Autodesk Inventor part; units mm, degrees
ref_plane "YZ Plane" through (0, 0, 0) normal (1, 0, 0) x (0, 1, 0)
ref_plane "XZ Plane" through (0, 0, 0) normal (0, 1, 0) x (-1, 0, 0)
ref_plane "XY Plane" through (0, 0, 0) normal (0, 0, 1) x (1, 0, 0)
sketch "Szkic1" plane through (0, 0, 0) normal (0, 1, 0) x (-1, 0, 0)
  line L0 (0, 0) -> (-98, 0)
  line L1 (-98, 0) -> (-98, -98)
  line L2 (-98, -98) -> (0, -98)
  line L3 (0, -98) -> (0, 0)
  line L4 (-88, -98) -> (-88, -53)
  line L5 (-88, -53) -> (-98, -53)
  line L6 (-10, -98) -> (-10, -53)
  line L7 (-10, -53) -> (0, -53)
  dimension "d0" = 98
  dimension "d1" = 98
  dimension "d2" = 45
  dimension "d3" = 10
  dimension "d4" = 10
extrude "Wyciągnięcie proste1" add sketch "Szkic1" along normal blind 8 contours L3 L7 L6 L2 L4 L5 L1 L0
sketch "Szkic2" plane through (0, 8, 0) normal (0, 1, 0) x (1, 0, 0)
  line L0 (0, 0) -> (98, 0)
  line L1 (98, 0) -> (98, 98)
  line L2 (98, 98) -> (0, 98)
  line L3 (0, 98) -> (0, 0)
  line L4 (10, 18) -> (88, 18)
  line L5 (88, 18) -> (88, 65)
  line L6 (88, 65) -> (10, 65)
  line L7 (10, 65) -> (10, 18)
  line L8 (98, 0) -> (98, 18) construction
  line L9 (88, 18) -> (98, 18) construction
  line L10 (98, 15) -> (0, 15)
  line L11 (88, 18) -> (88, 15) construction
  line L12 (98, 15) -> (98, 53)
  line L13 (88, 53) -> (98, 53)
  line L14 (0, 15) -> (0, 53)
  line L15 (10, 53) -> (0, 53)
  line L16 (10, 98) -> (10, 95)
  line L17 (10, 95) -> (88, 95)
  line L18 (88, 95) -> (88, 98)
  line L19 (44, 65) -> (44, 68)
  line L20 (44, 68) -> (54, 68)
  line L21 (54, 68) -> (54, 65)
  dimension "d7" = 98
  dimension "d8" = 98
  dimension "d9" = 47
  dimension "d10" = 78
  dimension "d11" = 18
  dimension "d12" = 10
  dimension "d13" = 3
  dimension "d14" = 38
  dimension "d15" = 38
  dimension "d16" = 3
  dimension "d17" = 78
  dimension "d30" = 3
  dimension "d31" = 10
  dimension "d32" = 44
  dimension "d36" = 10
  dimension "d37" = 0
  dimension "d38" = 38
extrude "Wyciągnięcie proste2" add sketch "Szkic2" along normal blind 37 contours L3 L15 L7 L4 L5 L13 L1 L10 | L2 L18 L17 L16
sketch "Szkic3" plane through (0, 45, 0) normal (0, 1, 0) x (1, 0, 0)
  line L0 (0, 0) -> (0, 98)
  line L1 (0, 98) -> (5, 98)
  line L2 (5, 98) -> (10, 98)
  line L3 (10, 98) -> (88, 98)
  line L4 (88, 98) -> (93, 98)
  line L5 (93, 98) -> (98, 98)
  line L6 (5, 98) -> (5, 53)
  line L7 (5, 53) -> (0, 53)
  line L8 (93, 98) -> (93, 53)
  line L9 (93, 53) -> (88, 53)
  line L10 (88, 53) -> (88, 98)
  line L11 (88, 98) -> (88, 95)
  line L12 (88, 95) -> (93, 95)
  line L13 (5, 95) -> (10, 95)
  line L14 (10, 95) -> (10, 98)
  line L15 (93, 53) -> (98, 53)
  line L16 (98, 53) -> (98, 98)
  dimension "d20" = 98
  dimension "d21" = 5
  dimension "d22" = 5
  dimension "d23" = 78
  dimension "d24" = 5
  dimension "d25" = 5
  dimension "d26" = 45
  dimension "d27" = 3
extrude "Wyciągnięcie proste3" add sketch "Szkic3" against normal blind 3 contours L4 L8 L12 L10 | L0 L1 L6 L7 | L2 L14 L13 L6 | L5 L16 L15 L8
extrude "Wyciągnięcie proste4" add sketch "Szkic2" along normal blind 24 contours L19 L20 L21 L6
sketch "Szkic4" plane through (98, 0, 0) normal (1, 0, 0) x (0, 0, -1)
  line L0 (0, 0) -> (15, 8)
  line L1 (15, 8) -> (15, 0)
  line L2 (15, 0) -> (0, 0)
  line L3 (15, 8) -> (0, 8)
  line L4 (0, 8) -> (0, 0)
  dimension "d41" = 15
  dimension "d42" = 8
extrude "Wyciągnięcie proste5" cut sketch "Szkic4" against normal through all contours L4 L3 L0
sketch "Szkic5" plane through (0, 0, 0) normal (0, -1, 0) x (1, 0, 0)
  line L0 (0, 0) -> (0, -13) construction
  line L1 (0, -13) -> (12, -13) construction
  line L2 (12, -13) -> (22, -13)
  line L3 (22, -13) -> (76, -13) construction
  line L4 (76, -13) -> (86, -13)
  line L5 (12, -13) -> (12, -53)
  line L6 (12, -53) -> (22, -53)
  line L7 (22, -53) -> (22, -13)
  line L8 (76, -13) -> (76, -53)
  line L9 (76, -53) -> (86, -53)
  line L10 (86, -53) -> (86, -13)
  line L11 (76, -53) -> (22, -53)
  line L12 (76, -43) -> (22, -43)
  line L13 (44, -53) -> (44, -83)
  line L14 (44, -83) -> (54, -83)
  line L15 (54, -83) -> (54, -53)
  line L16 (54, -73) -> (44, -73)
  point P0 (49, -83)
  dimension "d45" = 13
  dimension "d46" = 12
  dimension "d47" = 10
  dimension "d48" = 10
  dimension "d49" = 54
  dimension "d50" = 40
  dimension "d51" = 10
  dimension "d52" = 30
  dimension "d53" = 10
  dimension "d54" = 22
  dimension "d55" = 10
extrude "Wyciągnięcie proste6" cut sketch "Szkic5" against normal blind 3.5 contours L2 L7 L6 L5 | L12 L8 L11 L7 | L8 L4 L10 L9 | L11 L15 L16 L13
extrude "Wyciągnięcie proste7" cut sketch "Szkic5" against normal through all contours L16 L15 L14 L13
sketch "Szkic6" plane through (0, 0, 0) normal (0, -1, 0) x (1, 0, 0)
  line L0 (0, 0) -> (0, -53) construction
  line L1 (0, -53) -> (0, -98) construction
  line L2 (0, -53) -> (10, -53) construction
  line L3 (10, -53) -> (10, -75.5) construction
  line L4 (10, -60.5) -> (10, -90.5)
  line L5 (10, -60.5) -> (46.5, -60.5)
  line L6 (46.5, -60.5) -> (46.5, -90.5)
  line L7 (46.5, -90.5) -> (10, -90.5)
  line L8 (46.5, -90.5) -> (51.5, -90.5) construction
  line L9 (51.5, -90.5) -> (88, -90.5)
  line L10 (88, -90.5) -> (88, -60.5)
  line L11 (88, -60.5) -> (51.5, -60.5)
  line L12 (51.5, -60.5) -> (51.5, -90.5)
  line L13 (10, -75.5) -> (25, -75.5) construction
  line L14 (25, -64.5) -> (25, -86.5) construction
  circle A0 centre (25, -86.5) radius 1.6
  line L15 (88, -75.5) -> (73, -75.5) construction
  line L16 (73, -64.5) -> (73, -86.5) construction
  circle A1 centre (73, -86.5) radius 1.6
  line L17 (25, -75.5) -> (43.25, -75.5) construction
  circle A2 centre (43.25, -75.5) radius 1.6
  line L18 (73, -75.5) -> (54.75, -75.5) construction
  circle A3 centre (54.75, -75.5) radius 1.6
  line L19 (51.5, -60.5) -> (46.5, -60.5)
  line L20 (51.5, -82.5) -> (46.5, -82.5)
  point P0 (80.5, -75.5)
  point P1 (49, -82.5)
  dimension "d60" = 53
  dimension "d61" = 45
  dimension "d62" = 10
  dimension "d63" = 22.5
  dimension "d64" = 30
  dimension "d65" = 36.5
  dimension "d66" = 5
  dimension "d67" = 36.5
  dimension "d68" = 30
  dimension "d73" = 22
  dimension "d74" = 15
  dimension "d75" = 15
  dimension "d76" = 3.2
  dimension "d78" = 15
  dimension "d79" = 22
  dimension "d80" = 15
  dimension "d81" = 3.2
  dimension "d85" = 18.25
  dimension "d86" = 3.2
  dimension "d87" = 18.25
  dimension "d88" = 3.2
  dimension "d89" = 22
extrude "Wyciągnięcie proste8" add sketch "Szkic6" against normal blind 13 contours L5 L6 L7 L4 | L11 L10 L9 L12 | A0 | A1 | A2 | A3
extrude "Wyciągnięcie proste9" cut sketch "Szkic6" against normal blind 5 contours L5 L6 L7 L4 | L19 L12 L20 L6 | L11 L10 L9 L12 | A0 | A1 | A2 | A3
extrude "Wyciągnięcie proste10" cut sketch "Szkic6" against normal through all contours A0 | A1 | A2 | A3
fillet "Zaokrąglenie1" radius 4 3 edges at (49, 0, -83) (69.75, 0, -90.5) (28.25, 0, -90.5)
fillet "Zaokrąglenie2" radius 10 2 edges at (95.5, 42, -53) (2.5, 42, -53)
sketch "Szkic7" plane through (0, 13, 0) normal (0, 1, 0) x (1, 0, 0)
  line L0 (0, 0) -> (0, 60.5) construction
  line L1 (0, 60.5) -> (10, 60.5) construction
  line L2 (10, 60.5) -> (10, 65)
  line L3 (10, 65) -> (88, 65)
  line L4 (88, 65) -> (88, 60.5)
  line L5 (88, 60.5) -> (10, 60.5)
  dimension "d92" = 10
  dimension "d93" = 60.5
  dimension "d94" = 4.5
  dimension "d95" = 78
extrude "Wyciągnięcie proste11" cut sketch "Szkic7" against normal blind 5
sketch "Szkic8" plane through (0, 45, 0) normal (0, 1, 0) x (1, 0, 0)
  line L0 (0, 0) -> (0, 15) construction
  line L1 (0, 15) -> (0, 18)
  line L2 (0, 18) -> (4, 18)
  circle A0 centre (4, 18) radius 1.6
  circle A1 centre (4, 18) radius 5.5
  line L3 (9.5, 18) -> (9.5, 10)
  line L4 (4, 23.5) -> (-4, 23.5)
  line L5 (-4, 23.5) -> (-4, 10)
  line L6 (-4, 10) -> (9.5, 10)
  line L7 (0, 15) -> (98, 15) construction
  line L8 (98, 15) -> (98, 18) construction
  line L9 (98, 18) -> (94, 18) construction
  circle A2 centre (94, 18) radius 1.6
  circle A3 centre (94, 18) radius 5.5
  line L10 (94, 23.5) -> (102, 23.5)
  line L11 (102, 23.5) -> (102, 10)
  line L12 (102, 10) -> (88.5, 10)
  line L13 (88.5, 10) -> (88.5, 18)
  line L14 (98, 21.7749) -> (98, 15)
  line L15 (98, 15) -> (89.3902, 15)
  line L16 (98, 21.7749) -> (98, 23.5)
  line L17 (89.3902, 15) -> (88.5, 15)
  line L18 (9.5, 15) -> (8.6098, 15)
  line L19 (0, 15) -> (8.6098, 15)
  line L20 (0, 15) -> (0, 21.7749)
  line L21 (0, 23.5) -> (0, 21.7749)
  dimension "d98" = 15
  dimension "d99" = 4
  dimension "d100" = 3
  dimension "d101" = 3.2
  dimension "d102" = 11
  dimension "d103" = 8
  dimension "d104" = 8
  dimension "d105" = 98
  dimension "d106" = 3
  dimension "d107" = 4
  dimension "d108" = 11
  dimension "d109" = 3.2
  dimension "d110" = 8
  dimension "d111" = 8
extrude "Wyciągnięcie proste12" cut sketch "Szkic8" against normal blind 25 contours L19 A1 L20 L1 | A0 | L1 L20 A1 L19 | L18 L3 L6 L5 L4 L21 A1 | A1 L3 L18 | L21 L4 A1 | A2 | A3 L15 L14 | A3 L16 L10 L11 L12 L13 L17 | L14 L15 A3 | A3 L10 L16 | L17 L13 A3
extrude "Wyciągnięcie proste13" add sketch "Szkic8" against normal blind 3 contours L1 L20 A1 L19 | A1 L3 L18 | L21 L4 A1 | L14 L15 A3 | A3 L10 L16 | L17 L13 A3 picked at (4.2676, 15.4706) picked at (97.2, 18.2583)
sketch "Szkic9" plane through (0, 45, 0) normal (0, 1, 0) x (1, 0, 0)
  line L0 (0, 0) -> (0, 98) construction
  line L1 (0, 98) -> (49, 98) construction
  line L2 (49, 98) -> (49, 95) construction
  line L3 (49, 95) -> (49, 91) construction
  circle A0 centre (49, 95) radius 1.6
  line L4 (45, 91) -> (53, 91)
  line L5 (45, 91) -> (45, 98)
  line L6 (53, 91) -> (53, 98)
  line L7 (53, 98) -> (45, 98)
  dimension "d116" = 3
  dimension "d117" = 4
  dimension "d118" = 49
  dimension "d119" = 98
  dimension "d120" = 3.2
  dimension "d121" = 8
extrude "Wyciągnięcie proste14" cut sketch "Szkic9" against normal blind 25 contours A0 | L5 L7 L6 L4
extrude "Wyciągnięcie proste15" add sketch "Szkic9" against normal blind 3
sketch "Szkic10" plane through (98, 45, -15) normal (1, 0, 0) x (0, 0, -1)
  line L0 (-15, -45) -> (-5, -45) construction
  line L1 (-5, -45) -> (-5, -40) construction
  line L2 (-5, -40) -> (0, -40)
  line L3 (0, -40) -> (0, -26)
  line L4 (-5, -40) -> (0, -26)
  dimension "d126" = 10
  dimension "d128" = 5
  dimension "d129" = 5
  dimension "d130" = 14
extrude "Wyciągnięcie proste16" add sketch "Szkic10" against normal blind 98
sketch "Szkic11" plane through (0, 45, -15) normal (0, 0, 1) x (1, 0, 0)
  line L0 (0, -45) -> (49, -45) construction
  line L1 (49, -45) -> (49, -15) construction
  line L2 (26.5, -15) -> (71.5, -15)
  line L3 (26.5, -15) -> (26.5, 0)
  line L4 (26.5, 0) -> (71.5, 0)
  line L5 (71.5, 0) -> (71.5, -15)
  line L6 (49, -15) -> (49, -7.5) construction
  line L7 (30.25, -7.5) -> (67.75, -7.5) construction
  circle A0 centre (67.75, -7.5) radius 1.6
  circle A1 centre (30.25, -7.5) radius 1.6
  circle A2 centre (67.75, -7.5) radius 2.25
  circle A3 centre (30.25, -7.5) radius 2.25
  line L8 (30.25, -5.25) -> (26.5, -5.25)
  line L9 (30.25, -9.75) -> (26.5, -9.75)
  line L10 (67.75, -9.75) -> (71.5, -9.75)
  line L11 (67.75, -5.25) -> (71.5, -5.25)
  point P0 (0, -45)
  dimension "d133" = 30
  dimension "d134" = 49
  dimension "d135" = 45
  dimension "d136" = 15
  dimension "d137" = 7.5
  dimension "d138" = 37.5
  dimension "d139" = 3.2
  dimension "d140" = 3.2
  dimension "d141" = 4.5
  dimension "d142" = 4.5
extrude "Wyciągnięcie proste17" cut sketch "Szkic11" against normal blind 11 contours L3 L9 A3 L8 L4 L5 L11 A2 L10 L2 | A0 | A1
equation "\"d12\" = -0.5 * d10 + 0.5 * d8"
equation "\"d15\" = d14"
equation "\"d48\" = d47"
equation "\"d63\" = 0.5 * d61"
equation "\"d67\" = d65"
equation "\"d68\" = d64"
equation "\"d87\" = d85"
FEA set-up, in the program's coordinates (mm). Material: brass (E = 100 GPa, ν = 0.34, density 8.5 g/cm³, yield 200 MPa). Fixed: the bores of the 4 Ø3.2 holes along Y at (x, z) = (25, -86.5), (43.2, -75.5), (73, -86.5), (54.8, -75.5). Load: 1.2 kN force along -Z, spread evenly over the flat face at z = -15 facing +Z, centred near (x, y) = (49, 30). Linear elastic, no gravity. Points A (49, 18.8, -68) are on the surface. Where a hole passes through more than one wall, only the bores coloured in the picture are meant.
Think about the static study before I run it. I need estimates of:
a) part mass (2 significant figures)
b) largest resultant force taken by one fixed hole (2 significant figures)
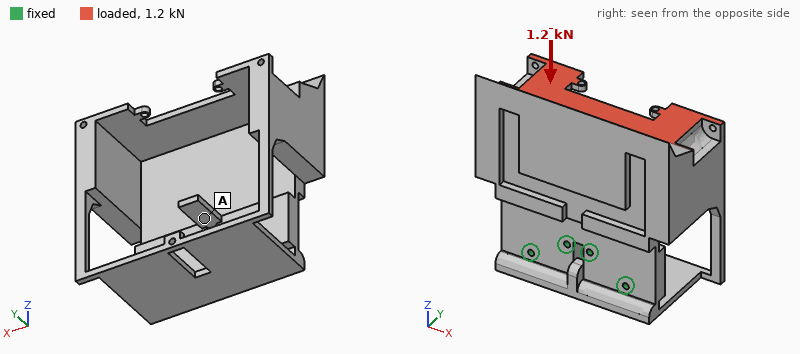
850 g
530 N
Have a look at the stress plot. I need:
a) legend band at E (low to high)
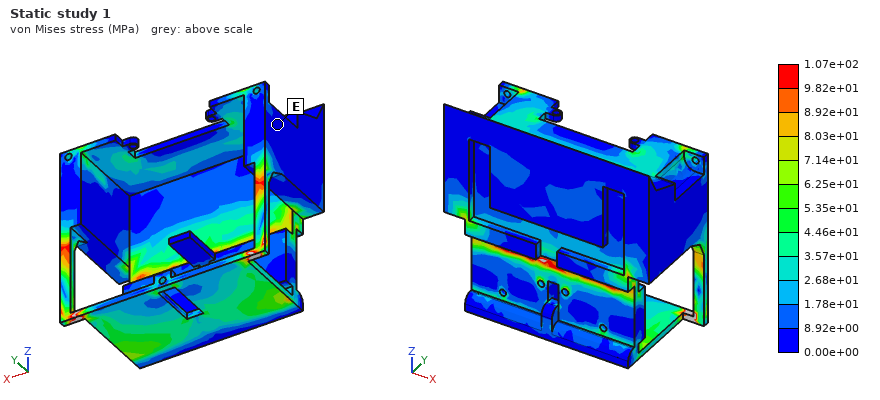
0.00e+00 to 8.92e+00 MPa
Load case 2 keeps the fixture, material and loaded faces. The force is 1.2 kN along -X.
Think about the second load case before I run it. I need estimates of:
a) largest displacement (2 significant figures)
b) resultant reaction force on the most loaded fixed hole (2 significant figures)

0.27 mm
1.4 kN
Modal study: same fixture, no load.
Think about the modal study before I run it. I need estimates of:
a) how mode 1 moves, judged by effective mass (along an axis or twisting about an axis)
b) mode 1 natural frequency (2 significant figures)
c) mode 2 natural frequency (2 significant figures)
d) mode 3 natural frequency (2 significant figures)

along Y
300 Hz
570 Hz
1600 Hz
